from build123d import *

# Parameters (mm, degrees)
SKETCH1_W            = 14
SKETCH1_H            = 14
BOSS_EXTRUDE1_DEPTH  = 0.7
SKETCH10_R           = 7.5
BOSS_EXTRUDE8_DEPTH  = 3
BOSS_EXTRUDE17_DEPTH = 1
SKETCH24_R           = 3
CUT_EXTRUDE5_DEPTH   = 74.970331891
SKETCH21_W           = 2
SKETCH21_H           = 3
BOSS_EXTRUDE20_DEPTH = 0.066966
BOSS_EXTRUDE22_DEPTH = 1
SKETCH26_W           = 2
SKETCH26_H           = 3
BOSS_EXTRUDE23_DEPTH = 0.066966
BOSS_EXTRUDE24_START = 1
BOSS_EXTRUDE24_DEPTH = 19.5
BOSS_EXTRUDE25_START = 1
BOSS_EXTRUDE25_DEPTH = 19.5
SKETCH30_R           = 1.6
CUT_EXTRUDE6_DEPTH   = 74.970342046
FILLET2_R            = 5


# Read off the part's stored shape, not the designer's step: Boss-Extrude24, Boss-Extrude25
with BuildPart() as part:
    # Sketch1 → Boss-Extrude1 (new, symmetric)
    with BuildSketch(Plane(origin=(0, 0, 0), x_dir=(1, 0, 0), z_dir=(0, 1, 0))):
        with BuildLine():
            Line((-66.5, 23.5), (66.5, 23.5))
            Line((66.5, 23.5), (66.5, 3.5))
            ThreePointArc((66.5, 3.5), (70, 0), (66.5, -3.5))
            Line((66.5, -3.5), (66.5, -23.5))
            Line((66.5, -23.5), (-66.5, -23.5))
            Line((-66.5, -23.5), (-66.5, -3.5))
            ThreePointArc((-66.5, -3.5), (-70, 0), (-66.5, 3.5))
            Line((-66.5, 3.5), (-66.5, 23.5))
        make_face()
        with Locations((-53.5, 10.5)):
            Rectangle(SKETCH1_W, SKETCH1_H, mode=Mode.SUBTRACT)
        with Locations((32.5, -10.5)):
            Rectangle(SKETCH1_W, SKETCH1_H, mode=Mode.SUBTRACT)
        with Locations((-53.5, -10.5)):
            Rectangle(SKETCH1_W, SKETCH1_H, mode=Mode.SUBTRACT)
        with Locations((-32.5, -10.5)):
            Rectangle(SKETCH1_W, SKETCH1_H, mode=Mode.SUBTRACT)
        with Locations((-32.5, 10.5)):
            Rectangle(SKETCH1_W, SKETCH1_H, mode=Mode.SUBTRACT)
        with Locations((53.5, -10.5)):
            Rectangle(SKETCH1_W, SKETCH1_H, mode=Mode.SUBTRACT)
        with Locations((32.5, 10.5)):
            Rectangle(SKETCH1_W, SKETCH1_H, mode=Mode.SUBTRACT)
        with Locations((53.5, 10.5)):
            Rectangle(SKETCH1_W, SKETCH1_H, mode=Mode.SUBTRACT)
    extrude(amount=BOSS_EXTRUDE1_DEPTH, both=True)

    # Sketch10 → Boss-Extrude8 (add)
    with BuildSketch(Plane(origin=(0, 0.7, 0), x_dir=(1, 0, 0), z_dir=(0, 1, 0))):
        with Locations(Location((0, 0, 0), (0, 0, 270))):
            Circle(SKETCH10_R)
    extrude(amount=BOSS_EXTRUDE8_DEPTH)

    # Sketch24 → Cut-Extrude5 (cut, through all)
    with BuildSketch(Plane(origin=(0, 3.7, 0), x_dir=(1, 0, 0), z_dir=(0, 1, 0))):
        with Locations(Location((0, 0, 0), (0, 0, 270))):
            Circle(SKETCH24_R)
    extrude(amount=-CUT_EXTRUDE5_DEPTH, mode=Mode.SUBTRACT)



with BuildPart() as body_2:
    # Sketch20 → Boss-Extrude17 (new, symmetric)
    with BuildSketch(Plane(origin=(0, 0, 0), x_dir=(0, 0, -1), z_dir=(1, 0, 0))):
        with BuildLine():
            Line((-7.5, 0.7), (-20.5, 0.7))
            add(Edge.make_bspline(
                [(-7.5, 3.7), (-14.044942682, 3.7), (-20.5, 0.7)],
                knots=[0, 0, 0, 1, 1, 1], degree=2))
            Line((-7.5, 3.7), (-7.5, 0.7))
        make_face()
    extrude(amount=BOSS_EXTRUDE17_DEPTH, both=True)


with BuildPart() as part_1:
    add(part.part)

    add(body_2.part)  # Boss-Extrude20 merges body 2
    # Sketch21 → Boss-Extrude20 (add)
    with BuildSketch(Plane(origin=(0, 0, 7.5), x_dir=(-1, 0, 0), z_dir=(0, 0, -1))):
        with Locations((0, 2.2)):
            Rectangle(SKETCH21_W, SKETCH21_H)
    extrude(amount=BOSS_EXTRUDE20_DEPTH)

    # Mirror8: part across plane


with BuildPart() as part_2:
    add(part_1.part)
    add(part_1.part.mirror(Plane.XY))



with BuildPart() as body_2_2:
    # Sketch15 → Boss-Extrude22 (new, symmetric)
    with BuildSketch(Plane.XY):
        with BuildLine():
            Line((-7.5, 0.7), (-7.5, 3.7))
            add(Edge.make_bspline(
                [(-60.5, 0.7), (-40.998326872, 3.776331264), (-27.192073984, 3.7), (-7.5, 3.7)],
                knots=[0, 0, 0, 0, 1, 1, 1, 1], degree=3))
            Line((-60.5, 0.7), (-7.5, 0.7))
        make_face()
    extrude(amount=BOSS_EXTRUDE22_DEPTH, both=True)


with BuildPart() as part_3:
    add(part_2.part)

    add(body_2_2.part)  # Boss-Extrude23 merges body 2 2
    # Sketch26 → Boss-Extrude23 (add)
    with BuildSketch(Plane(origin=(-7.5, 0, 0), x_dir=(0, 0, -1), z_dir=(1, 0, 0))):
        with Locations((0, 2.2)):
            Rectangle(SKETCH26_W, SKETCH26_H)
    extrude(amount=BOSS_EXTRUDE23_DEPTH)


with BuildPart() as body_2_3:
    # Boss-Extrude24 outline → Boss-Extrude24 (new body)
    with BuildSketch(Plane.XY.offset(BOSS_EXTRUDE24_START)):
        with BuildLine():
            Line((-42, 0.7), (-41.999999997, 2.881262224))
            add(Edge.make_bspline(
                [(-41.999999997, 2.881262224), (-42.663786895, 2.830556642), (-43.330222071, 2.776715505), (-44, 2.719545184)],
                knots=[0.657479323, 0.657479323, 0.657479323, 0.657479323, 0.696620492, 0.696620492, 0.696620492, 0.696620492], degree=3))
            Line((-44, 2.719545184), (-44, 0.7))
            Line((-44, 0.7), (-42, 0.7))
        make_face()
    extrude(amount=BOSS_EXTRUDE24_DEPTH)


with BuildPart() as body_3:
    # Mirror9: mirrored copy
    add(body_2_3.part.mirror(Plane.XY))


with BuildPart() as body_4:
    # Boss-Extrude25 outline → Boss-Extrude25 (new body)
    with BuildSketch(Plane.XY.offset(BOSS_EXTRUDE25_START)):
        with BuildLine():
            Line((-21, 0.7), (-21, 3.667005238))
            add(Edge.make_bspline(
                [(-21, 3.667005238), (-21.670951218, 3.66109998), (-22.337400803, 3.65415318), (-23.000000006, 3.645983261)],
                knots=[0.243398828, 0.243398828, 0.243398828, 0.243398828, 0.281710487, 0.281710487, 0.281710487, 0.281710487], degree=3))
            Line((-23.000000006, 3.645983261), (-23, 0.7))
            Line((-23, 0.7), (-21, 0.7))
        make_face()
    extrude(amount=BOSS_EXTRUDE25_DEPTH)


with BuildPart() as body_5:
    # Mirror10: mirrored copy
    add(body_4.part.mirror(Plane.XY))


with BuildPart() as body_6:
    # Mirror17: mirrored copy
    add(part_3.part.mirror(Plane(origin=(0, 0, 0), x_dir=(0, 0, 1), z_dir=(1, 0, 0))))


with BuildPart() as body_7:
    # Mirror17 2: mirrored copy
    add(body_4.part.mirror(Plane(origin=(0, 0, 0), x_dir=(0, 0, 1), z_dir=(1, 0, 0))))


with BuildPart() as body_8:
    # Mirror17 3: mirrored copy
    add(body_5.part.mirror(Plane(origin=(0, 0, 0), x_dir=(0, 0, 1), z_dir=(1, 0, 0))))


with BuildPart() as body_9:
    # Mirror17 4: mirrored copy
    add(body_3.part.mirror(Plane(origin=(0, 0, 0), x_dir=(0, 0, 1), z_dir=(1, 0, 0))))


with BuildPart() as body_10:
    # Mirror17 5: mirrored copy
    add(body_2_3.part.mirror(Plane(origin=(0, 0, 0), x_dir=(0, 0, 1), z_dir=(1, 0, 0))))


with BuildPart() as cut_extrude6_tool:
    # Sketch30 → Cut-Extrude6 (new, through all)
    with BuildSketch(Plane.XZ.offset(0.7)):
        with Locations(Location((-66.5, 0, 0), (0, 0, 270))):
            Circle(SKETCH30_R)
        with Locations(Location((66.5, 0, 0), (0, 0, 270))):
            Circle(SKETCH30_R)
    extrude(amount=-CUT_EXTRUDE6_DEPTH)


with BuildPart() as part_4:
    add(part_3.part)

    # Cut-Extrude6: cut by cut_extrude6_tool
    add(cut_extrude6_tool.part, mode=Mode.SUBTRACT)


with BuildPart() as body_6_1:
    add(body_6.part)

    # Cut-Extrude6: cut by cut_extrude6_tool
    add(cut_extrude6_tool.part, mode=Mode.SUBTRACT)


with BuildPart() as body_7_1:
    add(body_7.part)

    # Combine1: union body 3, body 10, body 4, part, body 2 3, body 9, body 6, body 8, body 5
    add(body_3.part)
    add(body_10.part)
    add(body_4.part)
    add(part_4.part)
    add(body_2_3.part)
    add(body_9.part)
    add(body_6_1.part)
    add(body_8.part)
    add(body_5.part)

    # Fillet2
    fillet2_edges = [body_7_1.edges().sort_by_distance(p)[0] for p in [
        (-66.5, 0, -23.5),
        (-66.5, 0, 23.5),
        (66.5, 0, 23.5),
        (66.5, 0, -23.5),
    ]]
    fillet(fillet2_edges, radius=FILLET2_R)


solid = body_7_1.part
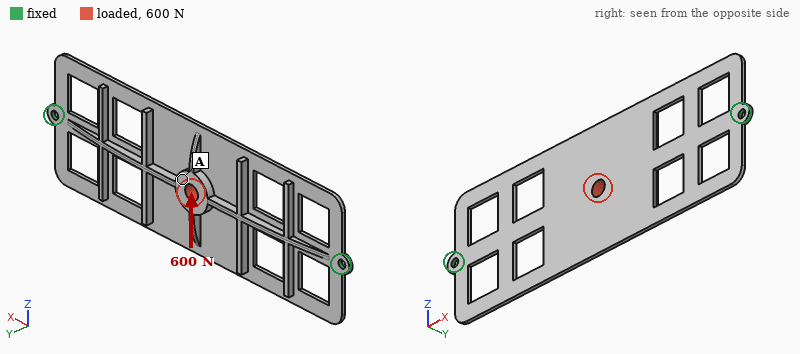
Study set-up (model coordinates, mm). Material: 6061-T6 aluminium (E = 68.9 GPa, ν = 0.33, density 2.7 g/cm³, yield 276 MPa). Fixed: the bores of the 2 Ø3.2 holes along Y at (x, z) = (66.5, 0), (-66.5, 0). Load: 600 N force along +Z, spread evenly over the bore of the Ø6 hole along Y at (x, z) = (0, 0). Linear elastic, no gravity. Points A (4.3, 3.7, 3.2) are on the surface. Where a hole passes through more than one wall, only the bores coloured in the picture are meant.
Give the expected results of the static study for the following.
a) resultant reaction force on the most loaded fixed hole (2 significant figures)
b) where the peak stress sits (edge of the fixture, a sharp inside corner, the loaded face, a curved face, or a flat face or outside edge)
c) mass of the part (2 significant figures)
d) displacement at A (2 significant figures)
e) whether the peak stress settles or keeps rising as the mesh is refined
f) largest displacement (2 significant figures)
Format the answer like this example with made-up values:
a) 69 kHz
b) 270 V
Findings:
a) 300 N
b) edge of the fixture
c) 23 g
d) 0.27 mm
e) keeps rising
f) 0.74 mm
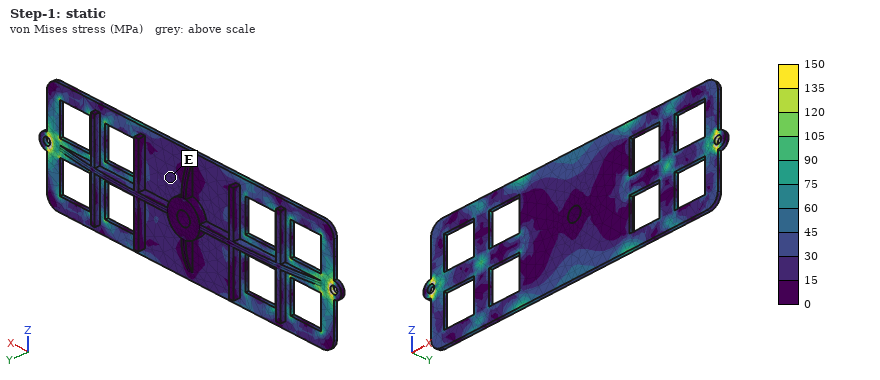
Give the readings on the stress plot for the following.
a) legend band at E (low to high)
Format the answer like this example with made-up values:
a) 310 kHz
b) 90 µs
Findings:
a) 15 to 30 MPa
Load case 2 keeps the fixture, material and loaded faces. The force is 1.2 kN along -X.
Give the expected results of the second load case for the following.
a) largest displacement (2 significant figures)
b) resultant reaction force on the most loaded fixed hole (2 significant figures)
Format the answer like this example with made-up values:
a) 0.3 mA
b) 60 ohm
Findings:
a) 43 µm
b) 600 N
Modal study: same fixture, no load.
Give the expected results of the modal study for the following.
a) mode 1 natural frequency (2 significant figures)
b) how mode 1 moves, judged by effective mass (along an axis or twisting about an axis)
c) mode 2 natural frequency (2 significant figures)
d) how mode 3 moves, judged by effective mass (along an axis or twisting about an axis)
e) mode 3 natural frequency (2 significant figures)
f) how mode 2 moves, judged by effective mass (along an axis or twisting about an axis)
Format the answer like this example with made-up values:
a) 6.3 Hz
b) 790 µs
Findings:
a) 440 Hz
b) along Y
c) 510 Hz
d) twisting about Z
e) 1300 Hz
f) twisting about X
